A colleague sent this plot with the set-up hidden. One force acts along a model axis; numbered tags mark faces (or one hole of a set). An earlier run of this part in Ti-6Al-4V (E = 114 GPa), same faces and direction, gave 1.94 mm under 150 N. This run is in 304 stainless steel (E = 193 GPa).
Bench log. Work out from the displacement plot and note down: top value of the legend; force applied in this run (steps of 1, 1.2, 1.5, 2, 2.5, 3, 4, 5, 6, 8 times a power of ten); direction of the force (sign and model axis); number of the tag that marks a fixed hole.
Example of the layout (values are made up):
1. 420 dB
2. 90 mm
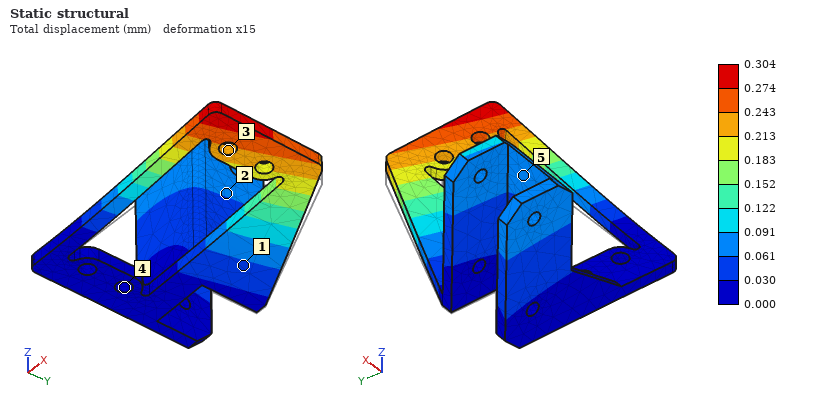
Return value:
1. 0.304 mm
2. 40 N
3. +Z
4. 4
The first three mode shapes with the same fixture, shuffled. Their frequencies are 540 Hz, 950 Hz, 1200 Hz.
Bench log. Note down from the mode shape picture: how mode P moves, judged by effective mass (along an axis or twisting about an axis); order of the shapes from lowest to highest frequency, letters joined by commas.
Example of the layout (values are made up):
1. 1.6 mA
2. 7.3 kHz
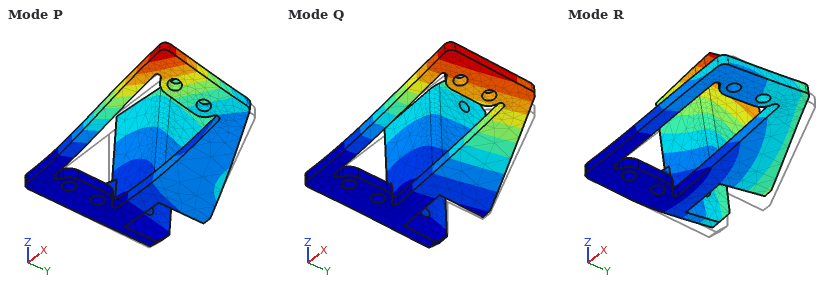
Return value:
1. along X
2. Q, R, P
